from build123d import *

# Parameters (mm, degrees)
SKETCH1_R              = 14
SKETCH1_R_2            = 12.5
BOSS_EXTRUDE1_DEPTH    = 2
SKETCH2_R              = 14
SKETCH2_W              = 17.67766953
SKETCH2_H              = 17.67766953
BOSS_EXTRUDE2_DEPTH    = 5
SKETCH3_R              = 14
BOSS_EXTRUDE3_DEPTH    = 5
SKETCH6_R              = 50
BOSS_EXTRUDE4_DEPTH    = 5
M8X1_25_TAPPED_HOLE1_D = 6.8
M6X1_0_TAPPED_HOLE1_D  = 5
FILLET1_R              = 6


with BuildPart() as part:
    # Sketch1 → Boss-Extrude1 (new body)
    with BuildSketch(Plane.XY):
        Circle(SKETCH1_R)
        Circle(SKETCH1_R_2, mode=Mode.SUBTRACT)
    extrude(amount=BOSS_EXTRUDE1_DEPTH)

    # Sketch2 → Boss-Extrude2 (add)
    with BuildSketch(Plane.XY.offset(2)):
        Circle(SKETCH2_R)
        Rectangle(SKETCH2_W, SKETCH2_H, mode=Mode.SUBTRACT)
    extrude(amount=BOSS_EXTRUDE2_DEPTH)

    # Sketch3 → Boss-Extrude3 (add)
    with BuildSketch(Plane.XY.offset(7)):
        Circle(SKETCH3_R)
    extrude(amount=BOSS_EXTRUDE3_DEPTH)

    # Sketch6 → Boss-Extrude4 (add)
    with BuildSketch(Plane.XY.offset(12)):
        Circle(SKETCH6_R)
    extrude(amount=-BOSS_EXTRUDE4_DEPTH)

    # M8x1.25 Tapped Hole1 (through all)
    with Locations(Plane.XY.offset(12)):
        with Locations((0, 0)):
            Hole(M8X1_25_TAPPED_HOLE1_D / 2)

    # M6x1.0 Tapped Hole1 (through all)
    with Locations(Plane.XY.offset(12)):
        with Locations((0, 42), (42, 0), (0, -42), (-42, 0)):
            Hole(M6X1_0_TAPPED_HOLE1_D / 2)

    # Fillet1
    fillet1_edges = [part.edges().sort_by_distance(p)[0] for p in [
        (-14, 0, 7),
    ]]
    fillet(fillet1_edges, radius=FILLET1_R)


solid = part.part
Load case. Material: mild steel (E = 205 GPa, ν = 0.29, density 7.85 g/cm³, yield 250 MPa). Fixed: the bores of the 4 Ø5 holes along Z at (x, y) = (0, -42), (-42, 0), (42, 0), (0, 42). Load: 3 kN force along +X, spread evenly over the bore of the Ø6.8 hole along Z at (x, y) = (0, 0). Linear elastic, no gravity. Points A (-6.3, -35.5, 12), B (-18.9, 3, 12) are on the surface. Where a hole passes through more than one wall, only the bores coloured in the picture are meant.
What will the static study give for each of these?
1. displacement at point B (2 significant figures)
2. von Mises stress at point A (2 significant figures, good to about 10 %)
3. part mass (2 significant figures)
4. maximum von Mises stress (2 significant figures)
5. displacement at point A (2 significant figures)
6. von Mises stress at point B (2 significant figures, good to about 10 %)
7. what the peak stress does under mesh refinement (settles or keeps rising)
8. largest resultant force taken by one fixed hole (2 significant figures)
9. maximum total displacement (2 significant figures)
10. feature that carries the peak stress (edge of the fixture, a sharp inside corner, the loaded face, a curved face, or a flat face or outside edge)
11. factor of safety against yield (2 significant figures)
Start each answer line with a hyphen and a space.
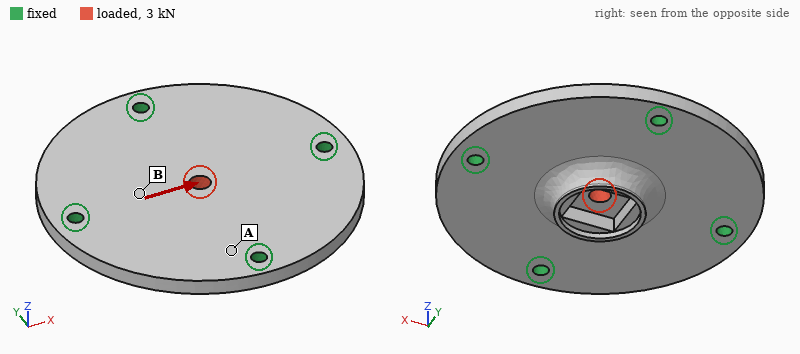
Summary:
- 1.2 µm
- 4.0 MPa
- 320 g
- 49 MPa
- 0.38 µm
- 11 MPa
- settles
- 960 N
- 2.5 µm
- the loaded face
- 5.1
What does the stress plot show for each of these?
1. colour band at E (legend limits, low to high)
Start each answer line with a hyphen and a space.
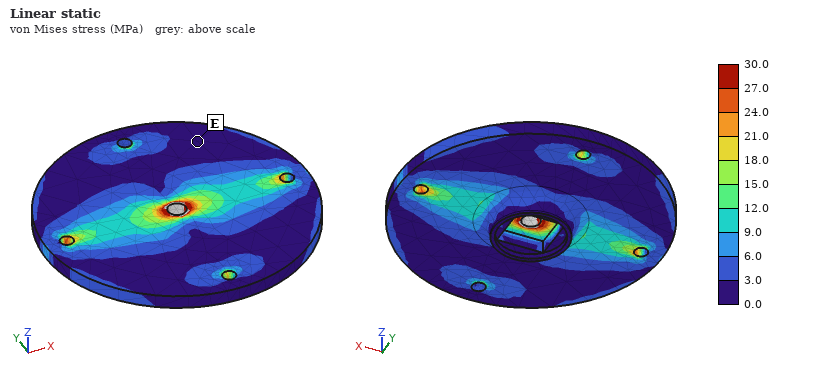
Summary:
- 0.0 to 3.0 MPa
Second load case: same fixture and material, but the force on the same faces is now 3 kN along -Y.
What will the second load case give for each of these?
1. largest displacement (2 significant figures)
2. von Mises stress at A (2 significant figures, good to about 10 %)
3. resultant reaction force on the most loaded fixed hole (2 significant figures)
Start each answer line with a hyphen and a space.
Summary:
- 2.5 µm
- 8.3 MPa
- 960 N
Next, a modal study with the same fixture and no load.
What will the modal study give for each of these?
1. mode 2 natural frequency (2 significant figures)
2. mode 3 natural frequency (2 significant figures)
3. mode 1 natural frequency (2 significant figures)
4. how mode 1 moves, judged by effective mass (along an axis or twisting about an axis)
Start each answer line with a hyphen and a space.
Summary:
- 5900 Hz
- 6100 Hz
- 5300 Hz
- along Z
